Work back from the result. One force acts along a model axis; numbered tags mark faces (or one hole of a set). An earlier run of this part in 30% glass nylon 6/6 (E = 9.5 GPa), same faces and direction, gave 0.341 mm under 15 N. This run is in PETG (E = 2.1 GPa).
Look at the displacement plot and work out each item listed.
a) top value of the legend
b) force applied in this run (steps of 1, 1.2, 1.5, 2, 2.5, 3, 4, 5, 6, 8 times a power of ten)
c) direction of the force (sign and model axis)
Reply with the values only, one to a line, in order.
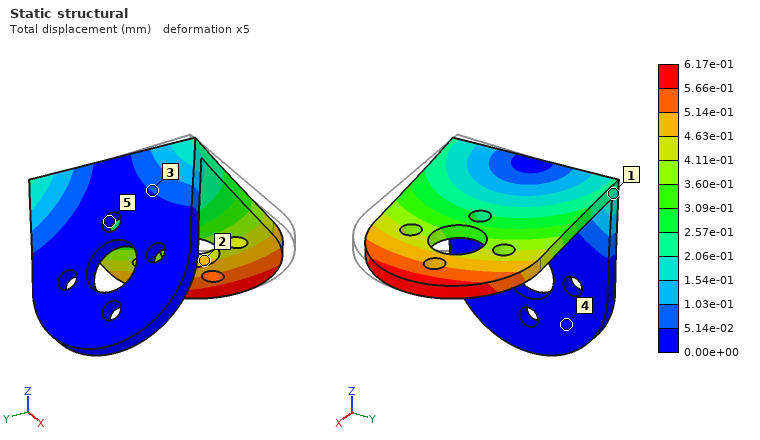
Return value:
6.17e-01 mm
6 N
+Y
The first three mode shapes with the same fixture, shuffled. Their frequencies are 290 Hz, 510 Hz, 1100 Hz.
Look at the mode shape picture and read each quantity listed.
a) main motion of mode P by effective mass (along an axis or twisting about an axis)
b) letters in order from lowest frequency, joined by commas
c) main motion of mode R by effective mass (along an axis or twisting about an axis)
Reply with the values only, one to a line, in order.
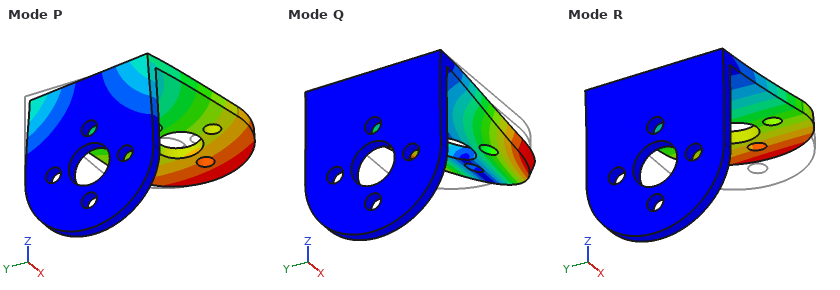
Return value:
along Y
R, P, Q
along Z
